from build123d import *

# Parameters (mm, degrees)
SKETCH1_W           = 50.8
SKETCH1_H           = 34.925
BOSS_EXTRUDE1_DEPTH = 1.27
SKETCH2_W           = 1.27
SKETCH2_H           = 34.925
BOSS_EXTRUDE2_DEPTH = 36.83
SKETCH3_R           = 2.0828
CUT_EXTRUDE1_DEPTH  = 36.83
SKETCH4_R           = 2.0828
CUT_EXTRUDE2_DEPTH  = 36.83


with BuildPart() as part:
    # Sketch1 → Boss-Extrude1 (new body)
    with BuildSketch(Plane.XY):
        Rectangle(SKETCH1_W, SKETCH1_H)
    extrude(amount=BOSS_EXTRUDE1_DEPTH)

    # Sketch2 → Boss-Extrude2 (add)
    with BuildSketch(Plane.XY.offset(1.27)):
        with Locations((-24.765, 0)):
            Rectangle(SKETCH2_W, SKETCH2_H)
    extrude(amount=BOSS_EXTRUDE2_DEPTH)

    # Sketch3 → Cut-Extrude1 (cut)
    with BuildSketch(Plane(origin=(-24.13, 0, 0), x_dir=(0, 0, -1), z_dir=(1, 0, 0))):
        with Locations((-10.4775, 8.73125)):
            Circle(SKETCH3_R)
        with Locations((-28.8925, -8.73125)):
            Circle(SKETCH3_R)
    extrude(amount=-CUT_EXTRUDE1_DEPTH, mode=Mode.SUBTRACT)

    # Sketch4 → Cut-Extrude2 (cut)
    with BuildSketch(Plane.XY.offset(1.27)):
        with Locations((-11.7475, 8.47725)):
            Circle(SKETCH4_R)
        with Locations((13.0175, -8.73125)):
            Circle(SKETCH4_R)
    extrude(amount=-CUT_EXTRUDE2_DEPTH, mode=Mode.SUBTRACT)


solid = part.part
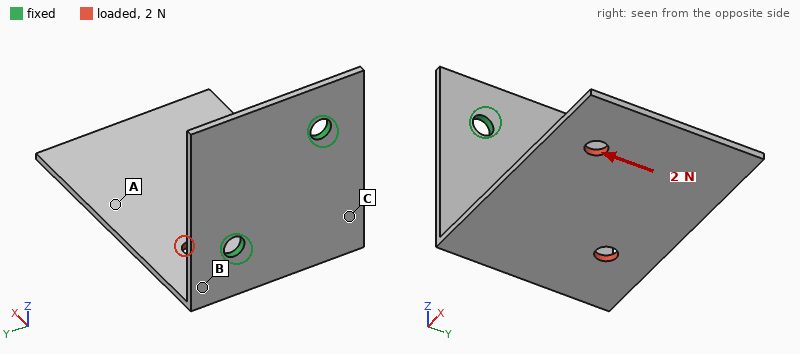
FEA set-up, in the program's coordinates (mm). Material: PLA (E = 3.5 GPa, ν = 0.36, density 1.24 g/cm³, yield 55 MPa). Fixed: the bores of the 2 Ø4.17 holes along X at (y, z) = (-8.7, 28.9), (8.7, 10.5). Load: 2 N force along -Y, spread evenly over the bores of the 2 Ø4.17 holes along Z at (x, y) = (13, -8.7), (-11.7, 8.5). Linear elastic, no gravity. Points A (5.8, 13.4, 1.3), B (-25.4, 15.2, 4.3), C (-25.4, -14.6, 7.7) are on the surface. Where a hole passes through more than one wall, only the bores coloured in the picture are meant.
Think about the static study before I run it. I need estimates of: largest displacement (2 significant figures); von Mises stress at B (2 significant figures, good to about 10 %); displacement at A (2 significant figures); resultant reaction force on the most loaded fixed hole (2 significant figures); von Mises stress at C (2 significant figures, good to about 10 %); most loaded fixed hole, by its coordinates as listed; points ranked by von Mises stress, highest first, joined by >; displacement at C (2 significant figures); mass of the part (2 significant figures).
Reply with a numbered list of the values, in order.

1. 0.77 mm
2. 2.3 MPa
3. 0.39 mm
4. 2.3 N
5. 1.4 MPa
6. (8.7, 10.5)
7. B > C > A
8. 0.19 mm
9. 4.7 g
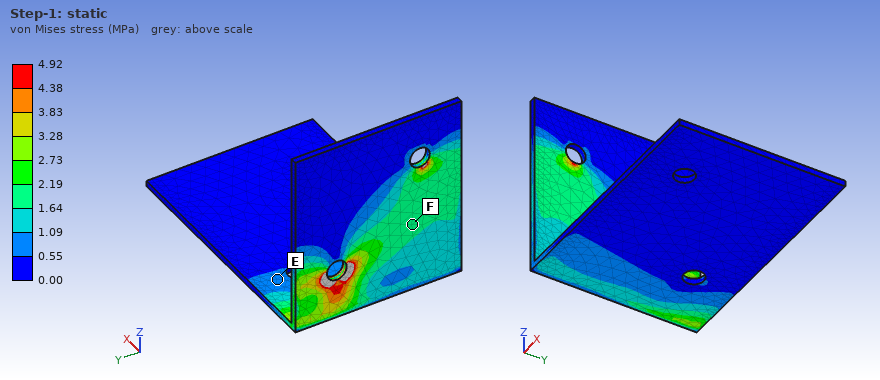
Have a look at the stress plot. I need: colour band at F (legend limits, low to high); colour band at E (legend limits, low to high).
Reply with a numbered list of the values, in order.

1. 1.64 to 2.19 MPa
2. 0.55 to 1.09 MPa
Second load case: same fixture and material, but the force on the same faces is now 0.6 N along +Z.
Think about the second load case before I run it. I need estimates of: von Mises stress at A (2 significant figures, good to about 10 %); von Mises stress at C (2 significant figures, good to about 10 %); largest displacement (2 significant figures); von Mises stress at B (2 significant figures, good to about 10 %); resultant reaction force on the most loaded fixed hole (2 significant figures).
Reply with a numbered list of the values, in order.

1. 0.29 MPa
2. 1.1 MPa
3. 0.83 mm
4. 1.6 MPa
5. 0.44 N
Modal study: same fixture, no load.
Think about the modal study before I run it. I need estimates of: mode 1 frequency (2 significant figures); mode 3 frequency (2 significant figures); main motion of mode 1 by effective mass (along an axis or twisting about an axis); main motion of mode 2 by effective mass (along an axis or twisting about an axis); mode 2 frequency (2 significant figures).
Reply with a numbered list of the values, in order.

1. 100 Hz
2. 420 Hz
3. along Z
4. along Y
5. 200 Hz
